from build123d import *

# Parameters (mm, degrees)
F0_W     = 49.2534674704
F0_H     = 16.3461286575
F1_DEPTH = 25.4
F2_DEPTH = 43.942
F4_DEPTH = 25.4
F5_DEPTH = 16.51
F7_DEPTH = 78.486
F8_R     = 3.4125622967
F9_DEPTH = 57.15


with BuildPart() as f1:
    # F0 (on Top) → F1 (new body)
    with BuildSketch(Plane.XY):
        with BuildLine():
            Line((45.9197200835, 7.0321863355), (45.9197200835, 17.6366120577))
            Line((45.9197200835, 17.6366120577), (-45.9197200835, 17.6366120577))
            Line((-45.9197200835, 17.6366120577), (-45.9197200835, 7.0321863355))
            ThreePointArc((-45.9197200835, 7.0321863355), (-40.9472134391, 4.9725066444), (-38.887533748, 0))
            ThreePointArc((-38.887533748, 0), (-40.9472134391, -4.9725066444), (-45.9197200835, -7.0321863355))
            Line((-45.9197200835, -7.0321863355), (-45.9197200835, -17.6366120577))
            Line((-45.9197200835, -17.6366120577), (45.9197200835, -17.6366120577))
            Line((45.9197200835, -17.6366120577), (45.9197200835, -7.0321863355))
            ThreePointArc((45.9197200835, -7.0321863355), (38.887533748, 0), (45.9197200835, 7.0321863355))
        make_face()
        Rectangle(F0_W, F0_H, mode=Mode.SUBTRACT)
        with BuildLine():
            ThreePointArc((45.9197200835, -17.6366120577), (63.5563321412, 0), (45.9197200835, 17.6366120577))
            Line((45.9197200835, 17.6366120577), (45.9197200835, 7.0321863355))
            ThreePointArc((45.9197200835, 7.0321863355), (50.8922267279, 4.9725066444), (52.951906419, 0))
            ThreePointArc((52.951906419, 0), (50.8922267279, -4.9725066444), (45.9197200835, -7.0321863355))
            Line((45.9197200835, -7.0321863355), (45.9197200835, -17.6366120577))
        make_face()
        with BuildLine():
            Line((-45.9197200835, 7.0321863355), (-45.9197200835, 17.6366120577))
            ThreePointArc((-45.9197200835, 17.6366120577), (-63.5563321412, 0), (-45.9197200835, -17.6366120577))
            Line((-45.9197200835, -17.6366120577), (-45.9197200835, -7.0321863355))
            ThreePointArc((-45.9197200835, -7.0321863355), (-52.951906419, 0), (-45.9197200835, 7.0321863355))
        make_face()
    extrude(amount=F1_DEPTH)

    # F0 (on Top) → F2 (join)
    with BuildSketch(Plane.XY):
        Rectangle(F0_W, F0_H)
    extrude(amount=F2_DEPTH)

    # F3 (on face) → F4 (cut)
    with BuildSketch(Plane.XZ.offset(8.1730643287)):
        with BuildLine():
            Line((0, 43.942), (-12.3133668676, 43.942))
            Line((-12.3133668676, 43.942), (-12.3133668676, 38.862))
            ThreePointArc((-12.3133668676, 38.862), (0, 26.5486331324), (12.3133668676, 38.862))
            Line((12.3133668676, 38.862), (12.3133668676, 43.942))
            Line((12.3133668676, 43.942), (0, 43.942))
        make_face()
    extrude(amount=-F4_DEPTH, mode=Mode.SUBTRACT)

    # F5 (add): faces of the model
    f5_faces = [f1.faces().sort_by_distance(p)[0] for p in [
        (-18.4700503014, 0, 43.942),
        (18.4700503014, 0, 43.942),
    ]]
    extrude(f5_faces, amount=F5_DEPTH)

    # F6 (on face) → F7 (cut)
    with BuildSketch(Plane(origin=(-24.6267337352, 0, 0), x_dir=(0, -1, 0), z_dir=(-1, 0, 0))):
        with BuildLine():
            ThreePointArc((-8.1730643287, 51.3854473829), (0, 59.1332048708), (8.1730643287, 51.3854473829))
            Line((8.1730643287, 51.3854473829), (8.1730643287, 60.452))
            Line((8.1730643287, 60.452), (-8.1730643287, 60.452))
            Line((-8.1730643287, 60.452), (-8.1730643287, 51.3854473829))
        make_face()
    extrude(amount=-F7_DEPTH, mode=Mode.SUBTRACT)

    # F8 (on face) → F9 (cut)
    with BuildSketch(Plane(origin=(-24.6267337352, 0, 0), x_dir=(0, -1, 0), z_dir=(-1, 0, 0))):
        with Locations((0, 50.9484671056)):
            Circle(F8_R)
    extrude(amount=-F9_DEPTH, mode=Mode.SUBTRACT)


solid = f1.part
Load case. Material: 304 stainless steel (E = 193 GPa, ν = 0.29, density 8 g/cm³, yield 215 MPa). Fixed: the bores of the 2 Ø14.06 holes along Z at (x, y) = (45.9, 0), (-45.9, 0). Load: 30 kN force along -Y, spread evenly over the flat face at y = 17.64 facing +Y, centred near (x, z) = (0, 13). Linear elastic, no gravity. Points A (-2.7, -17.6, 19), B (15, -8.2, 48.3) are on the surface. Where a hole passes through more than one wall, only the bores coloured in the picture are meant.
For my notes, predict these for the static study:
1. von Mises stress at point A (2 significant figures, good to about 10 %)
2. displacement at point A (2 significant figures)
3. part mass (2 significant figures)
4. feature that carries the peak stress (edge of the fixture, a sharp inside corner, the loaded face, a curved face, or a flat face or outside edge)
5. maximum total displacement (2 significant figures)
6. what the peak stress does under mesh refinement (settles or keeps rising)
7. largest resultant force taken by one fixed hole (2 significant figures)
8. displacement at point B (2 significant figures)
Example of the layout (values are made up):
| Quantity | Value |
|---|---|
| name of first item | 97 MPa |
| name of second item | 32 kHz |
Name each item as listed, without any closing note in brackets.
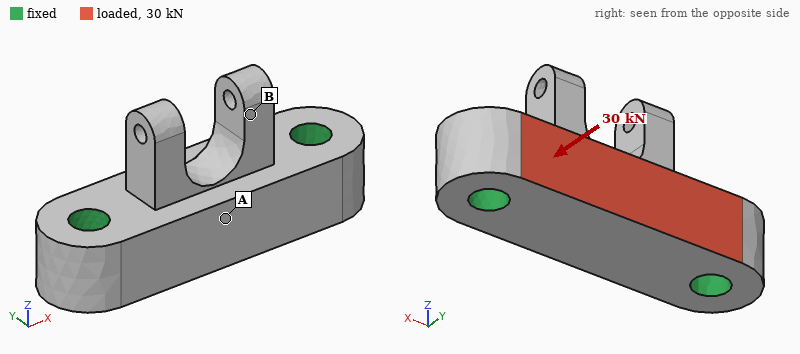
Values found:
| Quantity | Value |
|---|---|
| von Mises stress at point A | 29 MPa |
| displacement at point A | 8.7 µm |
| part mass | 900 g |
| feature that carries the peak stress | edge of the fixture |
| maximum total displacement | 10 µm |
| what the peak stress does under mesh refinement | keeps rising |
| largest resultant force taken by one fixed hole | 15 kN |
| displacement at point B | 8.7 µm |
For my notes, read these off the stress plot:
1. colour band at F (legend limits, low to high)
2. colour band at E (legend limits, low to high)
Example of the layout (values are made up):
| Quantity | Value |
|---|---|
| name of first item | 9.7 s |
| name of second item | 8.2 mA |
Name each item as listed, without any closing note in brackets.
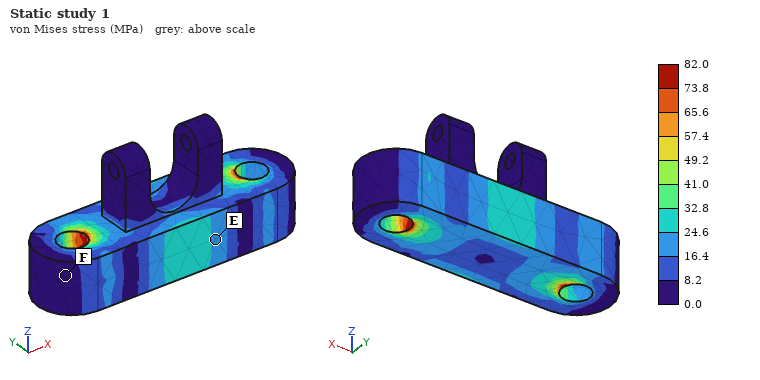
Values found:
| Quantity | Value |
|---|---|
| colour band at F | 0.0 to 8.2 MPa |
| colour band at E | 16.4 to 24.6 MPa |
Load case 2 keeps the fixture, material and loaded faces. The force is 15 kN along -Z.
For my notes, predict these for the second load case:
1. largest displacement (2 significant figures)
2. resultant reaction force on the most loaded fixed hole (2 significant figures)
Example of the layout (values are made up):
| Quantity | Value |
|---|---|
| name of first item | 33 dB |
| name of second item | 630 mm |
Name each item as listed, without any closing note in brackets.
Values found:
| Quantity | Value |
|---|---|
| largest displacement | 14 µm |
| resultant reaction force on the most loaded fixed hole | 7.5 kN |
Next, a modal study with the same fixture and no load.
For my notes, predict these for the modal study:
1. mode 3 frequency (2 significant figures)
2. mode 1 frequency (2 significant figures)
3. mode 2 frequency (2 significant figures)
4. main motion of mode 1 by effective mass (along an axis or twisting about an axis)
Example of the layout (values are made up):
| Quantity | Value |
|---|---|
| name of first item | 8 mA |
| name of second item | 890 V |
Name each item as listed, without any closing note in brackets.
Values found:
| Quantity | Value |
|---|---|
| mode 3 frequency | 9800 Hz |
| mode 1 frequency | 7700 Hz |
| mode 2 frequency | 9300 Hz |
| main motion of mode 1 by effective mass | along Y |
